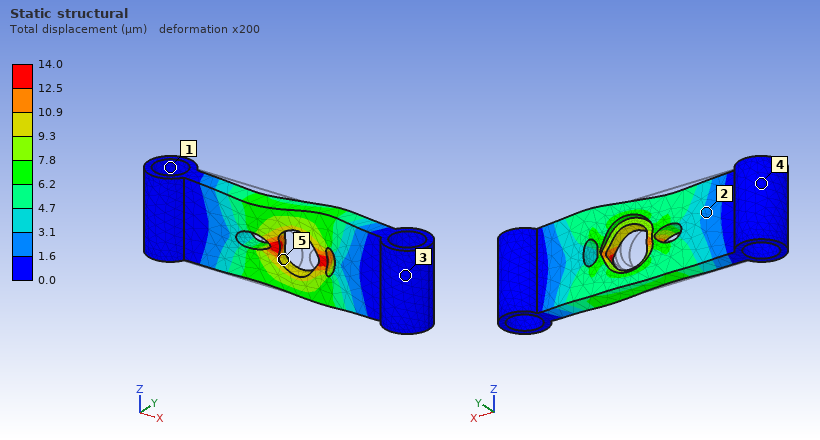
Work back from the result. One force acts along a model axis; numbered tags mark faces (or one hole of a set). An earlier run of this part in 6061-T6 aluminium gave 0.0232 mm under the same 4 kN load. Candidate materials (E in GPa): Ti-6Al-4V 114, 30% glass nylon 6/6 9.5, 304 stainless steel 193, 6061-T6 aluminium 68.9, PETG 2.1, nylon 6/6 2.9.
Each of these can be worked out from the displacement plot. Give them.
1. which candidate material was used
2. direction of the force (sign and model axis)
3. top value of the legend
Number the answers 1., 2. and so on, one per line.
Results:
1. Ti-6Al-4V
2. +X
3. 14.0 µm
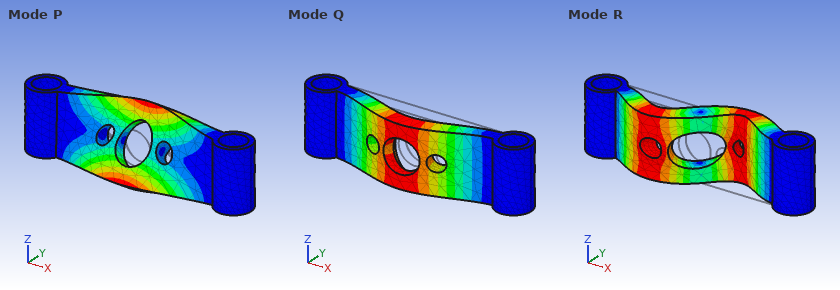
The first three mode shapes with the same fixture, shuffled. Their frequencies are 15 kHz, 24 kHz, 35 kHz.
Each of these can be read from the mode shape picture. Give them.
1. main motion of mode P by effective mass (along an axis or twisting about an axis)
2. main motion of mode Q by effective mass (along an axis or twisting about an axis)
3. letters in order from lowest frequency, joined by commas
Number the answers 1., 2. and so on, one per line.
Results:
1. twisting about X
2. along Y
3. Q, P, R
